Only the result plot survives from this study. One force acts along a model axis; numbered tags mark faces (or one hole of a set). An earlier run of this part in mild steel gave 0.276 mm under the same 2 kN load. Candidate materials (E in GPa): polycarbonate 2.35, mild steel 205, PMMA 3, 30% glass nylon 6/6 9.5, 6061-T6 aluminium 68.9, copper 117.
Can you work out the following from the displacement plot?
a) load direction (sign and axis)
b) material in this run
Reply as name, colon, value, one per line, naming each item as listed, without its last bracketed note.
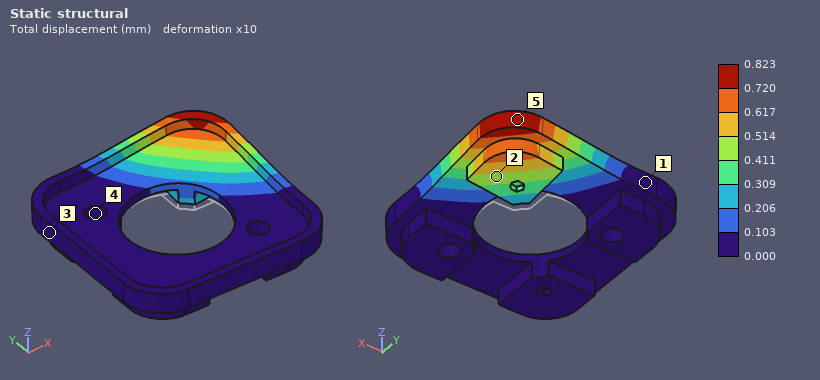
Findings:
load direction: +Z
material in this run: 6061-T6 aluminium
